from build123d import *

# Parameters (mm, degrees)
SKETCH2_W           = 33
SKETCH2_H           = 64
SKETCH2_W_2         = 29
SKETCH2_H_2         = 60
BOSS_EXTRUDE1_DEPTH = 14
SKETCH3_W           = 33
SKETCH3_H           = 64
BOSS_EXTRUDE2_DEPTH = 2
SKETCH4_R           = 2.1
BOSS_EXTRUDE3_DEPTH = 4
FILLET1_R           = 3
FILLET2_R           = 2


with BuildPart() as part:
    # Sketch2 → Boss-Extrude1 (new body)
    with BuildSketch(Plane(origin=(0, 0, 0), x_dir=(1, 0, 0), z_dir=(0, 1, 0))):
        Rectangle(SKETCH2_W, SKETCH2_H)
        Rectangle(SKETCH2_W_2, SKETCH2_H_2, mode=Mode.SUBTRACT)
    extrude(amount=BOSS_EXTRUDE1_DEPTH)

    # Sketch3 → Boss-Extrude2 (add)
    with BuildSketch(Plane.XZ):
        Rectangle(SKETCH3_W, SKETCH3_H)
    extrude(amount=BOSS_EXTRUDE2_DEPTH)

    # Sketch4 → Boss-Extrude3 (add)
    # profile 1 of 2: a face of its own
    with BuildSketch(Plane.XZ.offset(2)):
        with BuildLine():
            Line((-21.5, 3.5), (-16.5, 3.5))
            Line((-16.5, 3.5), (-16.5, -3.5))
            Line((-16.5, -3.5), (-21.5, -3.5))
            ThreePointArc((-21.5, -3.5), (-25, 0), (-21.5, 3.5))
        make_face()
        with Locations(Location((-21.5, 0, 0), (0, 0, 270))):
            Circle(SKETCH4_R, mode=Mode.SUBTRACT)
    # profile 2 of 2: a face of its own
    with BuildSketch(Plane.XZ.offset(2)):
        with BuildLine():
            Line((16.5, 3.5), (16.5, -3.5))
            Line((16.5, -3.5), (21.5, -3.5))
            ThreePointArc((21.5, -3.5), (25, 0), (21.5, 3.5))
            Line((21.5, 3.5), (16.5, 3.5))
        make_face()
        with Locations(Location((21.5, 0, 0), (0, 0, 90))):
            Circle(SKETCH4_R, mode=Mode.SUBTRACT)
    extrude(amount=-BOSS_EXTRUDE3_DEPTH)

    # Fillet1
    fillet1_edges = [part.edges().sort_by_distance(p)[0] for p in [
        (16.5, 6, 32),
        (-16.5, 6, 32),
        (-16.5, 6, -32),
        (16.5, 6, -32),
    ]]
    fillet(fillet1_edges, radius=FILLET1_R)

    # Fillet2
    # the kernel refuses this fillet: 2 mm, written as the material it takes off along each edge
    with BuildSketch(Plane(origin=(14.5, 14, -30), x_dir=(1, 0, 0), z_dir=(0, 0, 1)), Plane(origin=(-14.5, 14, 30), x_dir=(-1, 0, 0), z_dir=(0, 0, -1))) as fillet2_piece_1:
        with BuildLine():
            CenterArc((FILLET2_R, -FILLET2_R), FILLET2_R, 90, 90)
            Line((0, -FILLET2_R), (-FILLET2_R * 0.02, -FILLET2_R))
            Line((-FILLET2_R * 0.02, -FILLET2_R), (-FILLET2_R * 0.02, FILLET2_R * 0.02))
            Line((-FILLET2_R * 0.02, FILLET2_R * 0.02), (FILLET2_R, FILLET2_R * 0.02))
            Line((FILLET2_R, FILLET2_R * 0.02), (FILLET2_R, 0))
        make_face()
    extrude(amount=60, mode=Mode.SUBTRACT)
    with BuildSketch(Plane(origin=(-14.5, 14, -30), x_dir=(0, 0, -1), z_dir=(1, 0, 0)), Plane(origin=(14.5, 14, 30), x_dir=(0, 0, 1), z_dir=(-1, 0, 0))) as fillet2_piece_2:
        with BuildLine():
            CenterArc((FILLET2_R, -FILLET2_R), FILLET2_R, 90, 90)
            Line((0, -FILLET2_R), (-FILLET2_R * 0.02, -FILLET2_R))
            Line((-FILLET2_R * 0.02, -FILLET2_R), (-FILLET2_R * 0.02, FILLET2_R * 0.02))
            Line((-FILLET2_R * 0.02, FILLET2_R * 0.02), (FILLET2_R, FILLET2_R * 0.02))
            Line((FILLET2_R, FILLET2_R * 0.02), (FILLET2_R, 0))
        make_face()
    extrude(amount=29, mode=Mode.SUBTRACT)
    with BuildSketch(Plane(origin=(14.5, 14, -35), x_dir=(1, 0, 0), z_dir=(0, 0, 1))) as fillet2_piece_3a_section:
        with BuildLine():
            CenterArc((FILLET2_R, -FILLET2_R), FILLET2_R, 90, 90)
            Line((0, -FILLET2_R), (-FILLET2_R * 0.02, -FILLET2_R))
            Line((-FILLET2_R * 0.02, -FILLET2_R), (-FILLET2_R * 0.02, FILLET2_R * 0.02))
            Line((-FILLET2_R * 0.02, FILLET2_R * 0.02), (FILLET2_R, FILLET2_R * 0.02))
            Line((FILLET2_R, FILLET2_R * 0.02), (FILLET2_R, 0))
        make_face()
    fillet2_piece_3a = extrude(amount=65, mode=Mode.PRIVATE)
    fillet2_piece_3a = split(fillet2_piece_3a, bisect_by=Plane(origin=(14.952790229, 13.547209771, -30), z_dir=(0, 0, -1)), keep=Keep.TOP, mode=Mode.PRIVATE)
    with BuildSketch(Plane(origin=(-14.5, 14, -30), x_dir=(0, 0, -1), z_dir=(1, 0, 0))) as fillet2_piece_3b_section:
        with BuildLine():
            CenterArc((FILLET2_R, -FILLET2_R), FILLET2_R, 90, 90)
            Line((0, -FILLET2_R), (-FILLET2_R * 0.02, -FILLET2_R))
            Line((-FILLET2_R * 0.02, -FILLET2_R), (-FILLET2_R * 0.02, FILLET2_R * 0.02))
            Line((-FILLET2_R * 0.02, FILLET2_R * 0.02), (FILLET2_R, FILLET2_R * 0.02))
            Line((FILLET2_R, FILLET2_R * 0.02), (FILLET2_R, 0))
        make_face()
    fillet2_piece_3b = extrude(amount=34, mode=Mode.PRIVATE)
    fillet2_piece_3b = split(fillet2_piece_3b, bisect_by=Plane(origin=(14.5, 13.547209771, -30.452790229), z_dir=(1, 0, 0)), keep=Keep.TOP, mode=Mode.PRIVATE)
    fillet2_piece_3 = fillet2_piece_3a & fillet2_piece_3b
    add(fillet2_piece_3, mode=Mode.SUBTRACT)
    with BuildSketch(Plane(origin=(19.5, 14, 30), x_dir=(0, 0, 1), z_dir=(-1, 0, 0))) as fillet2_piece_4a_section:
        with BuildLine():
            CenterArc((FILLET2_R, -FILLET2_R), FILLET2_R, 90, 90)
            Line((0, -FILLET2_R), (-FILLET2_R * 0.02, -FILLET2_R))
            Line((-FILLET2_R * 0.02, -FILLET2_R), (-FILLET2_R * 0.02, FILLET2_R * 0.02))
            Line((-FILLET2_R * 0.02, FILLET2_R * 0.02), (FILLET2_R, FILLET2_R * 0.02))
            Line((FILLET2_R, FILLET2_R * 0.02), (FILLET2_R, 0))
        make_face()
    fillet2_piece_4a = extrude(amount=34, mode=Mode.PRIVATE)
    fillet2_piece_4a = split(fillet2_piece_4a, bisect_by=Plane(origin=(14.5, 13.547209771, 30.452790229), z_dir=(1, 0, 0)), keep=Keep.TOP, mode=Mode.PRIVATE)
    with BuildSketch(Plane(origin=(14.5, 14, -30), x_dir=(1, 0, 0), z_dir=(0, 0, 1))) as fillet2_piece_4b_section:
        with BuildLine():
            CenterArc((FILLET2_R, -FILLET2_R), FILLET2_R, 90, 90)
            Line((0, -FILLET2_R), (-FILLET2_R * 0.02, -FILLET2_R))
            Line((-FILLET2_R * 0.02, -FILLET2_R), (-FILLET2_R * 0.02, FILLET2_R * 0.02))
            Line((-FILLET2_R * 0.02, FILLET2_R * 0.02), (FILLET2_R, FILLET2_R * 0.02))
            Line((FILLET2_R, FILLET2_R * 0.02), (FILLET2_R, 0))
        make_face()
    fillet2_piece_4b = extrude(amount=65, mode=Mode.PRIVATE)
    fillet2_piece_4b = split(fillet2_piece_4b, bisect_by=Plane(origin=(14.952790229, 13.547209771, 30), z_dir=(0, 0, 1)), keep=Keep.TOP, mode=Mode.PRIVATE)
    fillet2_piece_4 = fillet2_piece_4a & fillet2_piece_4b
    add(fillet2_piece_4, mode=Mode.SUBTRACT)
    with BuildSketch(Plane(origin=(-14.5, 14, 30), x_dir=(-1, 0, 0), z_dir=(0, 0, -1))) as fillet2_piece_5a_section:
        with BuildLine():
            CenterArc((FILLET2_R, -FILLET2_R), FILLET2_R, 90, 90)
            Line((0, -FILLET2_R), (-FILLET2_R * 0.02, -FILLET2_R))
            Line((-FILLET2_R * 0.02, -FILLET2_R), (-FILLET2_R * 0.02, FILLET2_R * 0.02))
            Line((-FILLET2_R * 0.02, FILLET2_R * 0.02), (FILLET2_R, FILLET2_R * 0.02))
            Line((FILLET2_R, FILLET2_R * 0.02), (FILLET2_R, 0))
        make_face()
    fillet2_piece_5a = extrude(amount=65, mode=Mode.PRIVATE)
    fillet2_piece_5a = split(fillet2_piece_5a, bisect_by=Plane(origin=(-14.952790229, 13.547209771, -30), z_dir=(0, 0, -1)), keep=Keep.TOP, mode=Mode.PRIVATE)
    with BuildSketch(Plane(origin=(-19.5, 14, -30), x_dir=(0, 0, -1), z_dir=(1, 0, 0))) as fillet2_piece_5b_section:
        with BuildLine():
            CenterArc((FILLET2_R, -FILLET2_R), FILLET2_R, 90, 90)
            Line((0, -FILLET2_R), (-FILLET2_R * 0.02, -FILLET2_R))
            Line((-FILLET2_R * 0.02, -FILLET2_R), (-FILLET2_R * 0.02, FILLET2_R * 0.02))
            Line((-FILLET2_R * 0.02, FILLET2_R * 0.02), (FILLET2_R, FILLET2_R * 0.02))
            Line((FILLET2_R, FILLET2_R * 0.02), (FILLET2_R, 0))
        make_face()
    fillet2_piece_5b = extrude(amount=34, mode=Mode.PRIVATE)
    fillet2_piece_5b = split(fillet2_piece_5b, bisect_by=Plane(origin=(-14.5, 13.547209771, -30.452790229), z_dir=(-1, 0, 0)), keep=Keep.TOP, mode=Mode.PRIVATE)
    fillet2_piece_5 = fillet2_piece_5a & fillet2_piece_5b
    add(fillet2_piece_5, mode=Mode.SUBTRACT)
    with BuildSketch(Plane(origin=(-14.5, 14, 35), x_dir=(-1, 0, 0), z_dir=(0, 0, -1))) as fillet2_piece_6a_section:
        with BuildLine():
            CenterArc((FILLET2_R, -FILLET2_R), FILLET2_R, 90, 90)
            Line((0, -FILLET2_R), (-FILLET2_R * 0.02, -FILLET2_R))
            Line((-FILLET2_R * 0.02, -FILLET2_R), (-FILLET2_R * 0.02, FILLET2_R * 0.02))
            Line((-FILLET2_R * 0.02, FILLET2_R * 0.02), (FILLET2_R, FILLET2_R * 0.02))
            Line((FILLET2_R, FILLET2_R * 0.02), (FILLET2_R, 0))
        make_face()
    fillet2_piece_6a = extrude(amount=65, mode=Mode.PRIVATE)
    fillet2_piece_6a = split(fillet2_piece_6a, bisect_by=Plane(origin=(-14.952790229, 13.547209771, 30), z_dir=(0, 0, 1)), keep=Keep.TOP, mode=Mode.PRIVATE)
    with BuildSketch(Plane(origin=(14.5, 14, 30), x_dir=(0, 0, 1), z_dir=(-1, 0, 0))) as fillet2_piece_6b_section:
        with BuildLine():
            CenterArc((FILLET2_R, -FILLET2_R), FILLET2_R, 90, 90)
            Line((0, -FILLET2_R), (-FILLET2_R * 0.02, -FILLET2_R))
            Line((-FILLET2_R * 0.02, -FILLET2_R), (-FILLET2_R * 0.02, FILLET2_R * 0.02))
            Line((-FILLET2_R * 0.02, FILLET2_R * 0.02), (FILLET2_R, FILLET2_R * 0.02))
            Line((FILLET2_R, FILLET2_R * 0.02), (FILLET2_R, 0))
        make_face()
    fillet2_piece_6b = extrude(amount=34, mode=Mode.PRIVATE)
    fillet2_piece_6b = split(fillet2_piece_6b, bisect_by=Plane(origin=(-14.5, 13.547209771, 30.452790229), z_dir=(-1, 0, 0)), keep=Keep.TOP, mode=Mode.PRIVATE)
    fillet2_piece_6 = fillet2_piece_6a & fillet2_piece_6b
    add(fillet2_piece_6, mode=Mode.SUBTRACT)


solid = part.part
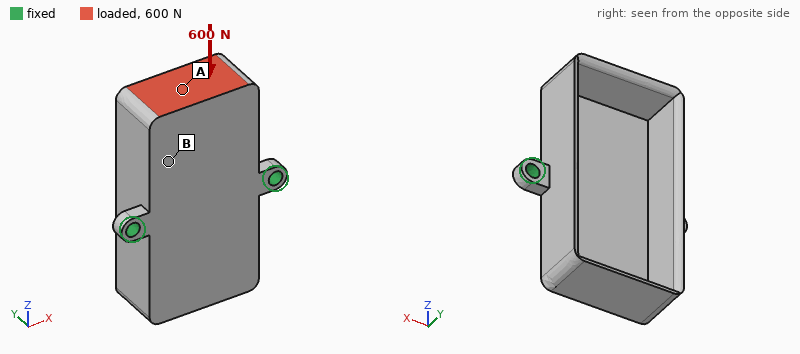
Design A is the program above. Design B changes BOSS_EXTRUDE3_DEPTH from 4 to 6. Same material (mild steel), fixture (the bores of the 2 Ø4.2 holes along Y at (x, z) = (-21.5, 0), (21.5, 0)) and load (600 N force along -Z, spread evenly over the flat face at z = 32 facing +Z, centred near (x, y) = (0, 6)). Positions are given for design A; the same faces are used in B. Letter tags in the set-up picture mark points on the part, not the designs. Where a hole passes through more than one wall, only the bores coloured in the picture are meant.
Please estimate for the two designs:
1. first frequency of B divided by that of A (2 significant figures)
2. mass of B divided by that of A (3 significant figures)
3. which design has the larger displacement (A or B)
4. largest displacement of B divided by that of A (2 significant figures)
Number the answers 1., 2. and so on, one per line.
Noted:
1. 1.4
2. 1.02
3. A
4. 0.71
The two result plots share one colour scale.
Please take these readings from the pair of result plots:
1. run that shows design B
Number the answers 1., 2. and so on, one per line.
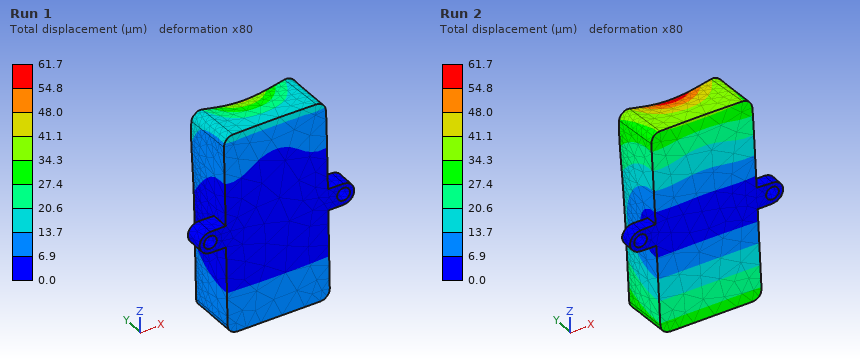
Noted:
1. Run 1
